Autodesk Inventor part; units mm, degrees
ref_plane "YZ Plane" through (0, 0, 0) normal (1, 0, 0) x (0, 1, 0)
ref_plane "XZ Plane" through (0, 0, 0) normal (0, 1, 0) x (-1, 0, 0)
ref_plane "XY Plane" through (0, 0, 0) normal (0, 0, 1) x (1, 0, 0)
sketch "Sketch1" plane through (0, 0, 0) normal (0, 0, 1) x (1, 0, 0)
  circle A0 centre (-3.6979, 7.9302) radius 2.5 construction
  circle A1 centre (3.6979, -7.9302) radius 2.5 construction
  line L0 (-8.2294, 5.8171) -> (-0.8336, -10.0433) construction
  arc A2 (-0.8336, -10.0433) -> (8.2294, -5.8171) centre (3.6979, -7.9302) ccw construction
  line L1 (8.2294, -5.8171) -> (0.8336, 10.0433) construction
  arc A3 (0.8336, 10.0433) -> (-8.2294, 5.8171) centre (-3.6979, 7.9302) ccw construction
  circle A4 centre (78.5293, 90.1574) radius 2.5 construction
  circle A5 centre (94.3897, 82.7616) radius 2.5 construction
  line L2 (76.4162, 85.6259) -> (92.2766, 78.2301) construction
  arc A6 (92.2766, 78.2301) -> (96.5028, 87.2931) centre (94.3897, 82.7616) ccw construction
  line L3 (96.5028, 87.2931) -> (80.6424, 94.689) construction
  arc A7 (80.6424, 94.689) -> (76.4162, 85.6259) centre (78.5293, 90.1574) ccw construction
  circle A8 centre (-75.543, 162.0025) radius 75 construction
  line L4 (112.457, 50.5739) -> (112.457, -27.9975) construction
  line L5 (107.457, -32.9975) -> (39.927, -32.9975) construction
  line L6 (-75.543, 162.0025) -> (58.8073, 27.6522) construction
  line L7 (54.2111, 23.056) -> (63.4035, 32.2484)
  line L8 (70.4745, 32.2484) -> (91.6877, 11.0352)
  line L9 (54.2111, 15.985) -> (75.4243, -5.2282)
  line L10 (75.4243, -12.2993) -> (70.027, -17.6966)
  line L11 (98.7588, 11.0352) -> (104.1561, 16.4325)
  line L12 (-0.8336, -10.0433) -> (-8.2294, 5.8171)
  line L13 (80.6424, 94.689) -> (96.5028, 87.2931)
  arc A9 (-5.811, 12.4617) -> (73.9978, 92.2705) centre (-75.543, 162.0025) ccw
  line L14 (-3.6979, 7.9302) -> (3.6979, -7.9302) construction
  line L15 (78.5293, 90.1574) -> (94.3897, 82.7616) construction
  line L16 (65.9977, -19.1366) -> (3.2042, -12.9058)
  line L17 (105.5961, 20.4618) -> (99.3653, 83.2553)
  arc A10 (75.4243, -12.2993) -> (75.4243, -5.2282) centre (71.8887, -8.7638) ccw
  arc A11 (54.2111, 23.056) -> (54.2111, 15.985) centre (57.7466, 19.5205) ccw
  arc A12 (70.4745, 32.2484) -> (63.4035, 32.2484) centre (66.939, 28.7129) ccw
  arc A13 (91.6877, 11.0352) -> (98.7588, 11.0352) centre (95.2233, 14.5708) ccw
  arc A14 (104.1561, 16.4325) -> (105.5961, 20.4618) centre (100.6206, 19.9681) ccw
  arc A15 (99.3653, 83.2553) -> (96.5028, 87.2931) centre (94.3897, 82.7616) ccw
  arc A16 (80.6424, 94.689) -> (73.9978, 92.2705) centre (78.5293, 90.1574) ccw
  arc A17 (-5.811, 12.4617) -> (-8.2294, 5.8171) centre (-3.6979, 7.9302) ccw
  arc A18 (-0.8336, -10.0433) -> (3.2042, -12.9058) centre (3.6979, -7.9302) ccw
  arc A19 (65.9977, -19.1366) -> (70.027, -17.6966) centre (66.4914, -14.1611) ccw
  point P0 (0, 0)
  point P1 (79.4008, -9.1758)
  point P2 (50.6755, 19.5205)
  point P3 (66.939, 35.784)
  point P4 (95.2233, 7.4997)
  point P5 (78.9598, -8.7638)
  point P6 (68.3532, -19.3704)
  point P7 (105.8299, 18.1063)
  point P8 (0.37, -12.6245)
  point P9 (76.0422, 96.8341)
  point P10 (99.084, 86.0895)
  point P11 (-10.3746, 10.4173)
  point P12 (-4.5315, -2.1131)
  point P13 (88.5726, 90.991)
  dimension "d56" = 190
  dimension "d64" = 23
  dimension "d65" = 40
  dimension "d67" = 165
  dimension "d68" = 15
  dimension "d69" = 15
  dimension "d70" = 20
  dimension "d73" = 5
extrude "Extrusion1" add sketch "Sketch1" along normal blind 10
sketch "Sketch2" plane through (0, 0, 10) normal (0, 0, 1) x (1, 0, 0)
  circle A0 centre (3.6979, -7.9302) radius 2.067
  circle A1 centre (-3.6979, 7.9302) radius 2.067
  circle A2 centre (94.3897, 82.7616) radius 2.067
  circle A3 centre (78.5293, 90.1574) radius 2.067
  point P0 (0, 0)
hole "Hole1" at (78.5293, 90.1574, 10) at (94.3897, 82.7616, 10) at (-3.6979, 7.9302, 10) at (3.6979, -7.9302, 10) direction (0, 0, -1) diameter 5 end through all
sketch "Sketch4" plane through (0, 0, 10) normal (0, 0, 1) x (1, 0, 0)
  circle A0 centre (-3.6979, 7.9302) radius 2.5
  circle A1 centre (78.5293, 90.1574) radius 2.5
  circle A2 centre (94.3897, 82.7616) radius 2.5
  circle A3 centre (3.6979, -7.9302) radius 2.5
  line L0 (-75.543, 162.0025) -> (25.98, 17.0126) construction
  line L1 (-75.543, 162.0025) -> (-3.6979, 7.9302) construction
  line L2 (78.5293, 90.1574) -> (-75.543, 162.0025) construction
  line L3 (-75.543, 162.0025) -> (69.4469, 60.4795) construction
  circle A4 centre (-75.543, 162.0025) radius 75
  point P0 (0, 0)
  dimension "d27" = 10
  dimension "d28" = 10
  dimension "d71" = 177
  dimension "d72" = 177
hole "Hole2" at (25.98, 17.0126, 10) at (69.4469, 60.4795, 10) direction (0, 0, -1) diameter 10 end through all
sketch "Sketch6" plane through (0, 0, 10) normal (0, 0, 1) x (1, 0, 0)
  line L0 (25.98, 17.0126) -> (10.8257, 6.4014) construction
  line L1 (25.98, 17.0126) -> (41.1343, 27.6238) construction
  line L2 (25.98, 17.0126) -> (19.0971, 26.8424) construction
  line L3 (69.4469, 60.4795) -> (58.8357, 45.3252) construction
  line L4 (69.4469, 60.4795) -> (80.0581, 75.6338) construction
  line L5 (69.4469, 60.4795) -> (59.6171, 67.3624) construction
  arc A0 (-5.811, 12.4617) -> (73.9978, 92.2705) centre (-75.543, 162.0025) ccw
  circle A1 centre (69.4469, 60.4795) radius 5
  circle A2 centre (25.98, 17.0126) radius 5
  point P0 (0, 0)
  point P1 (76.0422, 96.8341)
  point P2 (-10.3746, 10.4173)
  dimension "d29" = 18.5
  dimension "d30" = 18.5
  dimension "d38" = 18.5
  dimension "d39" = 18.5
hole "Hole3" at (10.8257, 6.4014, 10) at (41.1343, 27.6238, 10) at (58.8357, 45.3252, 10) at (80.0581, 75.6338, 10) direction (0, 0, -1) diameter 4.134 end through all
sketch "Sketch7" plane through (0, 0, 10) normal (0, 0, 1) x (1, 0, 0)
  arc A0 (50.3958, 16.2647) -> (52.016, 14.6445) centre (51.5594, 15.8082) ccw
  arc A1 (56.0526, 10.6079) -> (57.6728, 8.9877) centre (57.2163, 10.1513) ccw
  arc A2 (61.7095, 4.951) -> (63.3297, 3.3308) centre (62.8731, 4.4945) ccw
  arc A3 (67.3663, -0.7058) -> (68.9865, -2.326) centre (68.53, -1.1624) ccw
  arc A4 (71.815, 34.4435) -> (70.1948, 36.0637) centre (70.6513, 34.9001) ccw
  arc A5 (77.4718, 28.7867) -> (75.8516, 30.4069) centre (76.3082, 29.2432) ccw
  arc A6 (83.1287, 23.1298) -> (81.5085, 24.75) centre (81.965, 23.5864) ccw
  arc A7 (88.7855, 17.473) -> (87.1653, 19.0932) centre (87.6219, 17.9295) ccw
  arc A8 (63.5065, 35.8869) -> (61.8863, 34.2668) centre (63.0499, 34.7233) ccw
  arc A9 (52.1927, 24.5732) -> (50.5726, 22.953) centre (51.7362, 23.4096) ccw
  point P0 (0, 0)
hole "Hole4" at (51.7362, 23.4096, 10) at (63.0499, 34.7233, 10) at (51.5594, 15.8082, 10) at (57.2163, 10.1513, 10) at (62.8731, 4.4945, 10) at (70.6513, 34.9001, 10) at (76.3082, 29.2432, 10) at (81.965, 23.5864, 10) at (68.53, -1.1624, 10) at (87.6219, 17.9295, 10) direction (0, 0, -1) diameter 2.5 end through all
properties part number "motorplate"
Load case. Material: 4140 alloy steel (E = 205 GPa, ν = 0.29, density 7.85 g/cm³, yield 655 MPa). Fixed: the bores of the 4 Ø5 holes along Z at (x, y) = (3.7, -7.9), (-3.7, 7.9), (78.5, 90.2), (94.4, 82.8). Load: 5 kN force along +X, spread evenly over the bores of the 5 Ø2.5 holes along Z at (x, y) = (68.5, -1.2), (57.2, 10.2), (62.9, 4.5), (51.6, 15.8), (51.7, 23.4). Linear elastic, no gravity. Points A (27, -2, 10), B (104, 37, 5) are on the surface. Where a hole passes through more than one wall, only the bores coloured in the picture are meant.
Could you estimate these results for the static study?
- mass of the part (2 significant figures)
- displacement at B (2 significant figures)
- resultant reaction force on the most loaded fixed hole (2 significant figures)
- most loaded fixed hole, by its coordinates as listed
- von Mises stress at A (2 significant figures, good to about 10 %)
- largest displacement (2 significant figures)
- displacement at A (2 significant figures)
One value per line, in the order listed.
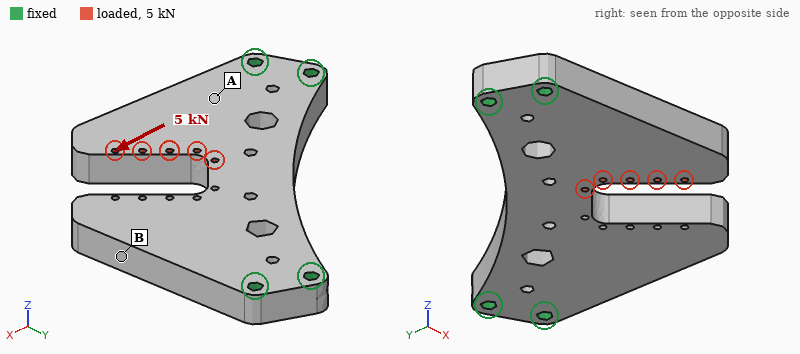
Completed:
470 g
5.1 µm
3.1 kN
(-3.7, 7.9)
12 MPa
11 µm
2.7 µm
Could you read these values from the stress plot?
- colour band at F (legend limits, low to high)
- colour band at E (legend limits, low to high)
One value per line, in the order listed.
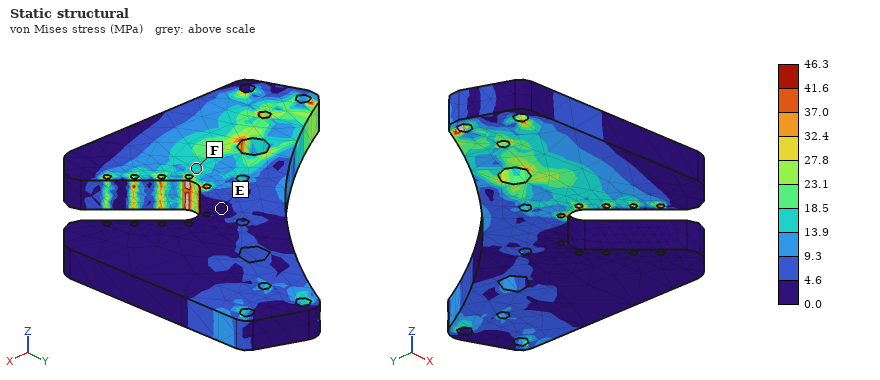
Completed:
13.9 to 18.5 MPa
0.0 to 4.6 MPa
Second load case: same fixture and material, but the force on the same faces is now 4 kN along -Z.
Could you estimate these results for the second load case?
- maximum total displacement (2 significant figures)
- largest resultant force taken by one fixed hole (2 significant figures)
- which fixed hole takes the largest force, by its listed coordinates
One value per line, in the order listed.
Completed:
0.33 mm
3.5 kN
(3.7, -7.9)
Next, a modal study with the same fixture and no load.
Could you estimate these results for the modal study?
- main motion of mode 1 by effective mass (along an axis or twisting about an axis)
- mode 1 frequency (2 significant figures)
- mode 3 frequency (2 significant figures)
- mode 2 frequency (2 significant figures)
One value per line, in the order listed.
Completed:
along Z
1800 Hz
4300 Hz
2900 Hz
